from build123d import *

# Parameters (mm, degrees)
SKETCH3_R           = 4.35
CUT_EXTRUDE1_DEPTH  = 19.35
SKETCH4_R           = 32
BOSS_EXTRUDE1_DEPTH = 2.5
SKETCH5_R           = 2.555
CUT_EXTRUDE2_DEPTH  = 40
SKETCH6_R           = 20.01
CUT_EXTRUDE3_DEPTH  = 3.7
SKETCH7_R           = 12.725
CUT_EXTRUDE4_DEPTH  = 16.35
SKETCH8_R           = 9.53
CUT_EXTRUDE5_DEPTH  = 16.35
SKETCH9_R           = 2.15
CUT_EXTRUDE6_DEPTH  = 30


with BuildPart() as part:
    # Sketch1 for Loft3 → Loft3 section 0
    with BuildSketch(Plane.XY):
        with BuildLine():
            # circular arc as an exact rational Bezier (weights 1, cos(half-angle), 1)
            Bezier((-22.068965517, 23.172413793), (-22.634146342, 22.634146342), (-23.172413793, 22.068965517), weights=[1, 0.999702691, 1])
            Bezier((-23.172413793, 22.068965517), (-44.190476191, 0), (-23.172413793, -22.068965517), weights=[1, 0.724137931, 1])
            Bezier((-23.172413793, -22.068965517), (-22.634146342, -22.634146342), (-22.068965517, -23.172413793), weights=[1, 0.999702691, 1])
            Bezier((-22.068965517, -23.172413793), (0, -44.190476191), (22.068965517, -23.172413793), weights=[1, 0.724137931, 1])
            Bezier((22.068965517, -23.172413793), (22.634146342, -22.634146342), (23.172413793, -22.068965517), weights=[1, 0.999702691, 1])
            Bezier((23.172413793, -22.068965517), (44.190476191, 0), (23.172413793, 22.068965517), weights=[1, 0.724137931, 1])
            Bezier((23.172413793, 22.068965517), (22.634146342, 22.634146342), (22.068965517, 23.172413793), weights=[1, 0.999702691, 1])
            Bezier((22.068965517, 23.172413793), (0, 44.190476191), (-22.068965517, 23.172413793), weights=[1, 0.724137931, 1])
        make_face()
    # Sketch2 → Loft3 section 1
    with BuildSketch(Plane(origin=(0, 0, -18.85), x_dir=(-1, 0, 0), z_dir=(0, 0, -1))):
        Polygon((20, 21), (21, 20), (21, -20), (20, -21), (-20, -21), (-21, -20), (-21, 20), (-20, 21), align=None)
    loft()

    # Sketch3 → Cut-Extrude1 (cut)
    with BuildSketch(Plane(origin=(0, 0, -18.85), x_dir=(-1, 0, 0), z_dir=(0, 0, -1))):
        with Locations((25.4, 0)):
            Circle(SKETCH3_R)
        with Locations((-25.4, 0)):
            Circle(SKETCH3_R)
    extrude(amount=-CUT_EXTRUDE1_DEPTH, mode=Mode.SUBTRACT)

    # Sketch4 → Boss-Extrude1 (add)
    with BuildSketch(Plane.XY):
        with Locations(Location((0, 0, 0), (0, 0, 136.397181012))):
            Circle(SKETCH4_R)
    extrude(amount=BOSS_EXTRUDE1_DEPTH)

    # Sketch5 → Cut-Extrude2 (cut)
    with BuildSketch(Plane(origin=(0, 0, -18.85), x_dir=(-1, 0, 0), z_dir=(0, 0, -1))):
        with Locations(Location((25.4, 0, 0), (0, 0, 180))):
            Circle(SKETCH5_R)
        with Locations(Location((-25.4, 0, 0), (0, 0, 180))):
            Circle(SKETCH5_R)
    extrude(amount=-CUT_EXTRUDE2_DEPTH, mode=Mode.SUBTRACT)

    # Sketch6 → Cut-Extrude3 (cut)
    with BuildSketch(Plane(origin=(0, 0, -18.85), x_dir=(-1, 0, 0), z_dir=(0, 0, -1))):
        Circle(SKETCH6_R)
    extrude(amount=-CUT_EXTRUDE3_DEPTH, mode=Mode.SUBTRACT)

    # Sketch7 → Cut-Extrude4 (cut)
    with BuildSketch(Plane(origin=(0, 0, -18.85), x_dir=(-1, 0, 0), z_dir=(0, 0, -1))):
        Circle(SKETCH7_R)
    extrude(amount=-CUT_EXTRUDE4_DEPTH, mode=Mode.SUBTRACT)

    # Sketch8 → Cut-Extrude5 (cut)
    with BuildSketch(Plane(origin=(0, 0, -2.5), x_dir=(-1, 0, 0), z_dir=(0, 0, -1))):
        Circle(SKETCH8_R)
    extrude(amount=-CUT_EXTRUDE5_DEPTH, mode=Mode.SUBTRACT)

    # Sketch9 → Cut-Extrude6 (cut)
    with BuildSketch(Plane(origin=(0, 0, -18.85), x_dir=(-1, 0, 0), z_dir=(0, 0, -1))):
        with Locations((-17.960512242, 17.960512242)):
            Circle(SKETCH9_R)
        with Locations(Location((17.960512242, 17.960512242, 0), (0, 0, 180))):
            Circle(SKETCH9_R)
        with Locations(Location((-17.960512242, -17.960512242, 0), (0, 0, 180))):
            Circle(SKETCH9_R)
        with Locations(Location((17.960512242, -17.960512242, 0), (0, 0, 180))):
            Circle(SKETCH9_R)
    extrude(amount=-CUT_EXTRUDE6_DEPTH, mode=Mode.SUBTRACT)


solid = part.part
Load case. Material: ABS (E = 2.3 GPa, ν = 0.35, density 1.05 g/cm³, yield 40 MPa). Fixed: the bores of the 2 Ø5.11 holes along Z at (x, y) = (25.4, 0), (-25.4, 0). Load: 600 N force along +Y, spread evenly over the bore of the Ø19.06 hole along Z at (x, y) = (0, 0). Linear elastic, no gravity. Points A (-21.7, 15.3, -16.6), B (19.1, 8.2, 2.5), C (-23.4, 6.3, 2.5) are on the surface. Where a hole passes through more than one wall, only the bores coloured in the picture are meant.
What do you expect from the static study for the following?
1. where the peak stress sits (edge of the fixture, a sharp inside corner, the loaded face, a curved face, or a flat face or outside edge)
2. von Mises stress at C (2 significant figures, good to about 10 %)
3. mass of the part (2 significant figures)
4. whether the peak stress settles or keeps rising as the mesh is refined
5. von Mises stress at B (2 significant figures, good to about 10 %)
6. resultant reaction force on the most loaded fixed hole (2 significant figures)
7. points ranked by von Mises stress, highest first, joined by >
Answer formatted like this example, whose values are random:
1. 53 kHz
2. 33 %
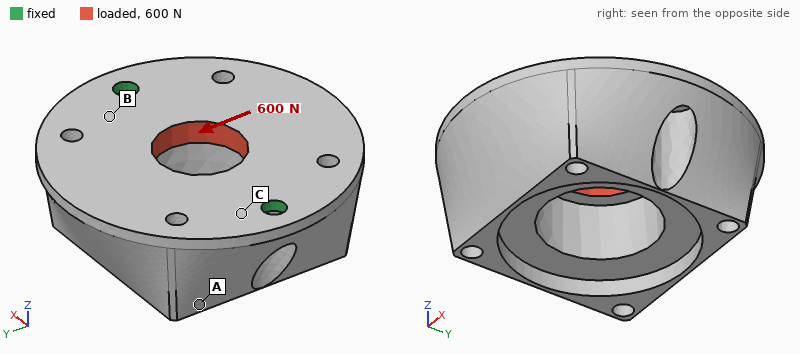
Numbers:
1. edge of the fixture
2. 5.0 MPa
3. 41 g
4. keeps rising
5. 2.6 MPa
6. 300 N
7. C > B > A
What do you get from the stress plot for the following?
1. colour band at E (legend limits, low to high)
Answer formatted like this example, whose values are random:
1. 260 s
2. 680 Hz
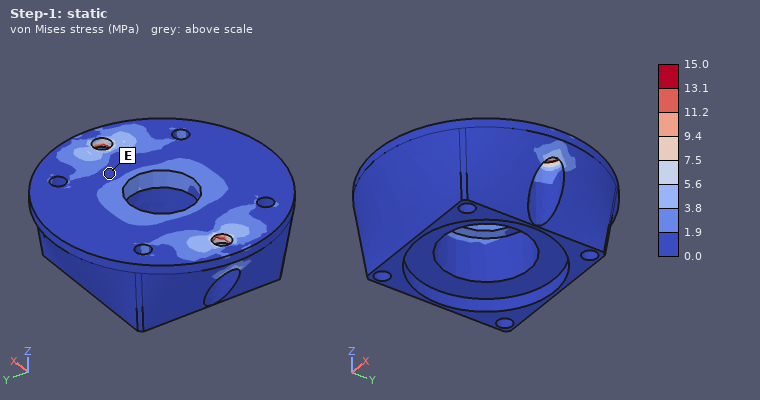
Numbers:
1. 0.0 to 1.9 MPa
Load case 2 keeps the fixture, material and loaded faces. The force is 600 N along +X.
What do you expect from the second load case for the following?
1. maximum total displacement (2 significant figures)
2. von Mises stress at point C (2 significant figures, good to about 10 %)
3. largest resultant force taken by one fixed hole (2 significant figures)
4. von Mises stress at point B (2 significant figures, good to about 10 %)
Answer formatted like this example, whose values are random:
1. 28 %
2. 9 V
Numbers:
1. 37 µm
2. 2.5 MPa
3. 300 N
4. 2.3 MPa
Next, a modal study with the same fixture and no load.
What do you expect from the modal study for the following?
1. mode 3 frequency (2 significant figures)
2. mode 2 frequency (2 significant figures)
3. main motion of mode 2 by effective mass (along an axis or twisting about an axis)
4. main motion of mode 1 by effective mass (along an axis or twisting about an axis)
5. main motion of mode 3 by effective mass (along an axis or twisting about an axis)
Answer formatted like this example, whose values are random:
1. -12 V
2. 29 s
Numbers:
1. 3400 Hz
2. 2400 Hz
3. along Z
4. along Y
5. along X
